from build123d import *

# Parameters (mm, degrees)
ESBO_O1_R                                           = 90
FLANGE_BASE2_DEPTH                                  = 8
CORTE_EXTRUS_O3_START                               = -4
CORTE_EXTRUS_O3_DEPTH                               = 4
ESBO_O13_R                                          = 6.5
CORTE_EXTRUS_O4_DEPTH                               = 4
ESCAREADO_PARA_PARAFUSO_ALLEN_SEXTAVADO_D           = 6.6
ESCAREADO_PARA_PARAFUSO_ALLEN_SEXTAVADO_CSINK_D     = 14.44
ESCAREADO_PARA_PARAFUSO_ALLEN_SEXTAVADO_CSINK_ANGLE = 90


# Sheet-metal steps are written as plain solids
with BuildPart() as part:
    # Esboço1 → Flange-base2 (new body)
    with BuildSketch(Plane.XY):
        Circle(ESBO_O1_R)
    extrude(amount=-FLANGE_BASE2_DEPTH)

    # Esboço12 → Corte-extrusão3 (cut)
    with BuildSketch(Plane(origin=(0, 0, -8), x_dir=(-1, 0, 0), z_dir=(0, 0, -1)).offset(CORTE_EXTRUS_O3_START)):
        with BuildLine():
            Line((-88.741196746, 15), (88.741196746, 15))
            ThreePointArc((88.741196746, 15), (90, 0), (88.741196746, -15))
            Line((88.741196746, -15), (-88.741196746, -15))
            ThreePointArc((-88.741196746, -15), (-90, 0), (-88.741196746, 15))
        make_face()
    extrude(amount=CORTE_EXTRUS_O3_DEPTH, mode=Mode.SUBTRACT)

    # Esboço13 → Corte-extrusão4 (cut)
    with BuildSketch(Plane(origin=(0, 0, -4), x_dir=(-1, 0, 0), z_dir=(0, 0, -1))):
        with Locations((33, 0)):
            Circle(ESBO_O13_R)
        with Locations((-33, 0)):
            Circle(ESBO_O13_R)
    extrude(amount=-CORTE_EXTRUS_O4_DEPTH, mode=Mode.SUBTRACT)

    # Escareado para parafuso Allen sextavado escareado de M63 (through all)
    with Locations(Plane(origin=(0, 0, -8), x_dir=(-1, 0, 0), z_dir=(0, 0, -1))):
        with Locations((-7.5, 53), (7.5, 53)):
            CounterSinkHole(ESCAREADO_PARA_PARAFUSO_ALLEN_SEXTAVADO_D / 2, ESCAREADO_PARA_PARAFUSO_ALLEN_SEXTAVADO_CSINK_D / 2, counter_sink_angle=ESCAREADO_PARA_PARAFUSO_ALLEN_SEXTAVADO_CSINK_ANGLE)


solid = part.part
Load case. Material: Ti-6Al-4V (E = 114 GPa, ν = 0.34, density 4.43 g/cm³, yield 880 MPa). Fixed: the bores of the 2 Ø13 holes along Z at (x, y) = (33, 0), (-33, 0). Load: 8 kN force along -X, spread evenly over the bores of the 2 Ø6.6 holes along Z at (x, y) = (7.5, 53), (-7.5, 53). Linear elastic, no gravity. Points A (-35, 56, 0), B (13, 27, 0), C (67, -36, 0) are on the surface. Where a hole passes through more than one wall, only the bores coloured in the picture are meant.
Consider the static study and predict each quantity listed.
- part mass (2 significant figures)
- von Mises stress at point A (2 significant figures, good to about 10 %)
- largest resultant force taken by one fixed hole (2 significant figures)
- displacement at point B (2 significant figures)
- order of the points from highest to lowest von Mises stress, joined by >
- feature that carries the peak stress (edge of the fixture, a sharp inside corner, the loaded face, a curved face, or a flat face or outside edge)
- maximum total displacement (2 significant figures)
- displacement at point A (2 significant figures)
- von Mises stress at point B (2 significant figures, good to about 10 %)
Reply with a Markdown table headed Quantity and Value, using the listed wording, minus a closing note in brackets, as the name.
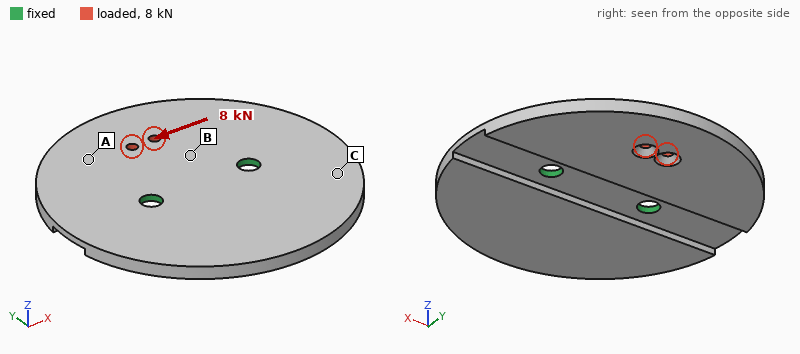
| Quantity | Value |
|---|---|
| part mass | 800 g |
| von Mises stress at point A | 16 MPa |
| largest resultant force taken by one fixed hole | 7.0 kN |
| displacement at point B | 15 µm |
| order of the points from highest to lowest von Mises stress, joined by > | B > A > C |
| feature that carries the peak stress | edge of the fixture |
| maximum total displacement | 63 µm |
| displacement at point A | 41 µm |
| von Mises stress at point B | 35 MPa |
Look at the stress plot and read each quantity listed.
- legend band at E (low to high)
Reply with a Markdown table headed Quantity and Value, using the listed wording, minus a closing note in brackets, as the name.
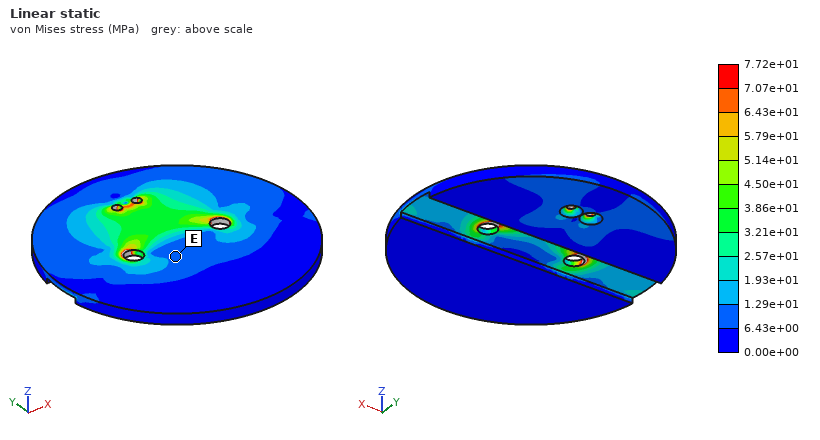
| Quantity | Value |
|---|---|
| legend band at E | 6.43e+00 to 1.29e+01 MPa |
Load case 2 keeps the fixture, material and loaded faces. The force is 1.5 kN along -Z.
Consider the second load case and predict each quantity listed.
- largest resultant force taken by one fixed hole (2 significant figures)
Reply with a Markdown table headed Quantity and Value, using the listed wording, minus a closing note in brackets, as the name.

| Quantity | Value |
|---|---|
| largest resultant force taken by one fixed hole | 790 N |
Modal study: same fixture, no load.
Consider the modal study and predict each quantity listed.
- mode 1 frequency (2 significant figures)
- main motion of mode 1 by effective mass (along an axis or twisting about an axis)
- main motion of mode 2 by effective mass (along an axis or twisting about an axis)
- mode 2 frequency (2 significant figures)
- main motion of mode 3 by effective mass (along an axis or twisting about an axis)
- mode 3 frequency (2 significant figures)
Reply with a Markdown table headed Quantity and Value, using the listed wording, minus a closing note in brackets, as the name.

| Quantity | Value |
|---|---|
| mode 1 frequency | 460 Hz |
| main motion of mode 1 by effective mass | twisting about X |
| main motion of mode 2 by effective mass | along Z |
| mode 2 frequency | 550 Hz |
| main motion of mode 3 by effective mass | twisting about Y |
| mode 3 frequency | 1100 Hz |
